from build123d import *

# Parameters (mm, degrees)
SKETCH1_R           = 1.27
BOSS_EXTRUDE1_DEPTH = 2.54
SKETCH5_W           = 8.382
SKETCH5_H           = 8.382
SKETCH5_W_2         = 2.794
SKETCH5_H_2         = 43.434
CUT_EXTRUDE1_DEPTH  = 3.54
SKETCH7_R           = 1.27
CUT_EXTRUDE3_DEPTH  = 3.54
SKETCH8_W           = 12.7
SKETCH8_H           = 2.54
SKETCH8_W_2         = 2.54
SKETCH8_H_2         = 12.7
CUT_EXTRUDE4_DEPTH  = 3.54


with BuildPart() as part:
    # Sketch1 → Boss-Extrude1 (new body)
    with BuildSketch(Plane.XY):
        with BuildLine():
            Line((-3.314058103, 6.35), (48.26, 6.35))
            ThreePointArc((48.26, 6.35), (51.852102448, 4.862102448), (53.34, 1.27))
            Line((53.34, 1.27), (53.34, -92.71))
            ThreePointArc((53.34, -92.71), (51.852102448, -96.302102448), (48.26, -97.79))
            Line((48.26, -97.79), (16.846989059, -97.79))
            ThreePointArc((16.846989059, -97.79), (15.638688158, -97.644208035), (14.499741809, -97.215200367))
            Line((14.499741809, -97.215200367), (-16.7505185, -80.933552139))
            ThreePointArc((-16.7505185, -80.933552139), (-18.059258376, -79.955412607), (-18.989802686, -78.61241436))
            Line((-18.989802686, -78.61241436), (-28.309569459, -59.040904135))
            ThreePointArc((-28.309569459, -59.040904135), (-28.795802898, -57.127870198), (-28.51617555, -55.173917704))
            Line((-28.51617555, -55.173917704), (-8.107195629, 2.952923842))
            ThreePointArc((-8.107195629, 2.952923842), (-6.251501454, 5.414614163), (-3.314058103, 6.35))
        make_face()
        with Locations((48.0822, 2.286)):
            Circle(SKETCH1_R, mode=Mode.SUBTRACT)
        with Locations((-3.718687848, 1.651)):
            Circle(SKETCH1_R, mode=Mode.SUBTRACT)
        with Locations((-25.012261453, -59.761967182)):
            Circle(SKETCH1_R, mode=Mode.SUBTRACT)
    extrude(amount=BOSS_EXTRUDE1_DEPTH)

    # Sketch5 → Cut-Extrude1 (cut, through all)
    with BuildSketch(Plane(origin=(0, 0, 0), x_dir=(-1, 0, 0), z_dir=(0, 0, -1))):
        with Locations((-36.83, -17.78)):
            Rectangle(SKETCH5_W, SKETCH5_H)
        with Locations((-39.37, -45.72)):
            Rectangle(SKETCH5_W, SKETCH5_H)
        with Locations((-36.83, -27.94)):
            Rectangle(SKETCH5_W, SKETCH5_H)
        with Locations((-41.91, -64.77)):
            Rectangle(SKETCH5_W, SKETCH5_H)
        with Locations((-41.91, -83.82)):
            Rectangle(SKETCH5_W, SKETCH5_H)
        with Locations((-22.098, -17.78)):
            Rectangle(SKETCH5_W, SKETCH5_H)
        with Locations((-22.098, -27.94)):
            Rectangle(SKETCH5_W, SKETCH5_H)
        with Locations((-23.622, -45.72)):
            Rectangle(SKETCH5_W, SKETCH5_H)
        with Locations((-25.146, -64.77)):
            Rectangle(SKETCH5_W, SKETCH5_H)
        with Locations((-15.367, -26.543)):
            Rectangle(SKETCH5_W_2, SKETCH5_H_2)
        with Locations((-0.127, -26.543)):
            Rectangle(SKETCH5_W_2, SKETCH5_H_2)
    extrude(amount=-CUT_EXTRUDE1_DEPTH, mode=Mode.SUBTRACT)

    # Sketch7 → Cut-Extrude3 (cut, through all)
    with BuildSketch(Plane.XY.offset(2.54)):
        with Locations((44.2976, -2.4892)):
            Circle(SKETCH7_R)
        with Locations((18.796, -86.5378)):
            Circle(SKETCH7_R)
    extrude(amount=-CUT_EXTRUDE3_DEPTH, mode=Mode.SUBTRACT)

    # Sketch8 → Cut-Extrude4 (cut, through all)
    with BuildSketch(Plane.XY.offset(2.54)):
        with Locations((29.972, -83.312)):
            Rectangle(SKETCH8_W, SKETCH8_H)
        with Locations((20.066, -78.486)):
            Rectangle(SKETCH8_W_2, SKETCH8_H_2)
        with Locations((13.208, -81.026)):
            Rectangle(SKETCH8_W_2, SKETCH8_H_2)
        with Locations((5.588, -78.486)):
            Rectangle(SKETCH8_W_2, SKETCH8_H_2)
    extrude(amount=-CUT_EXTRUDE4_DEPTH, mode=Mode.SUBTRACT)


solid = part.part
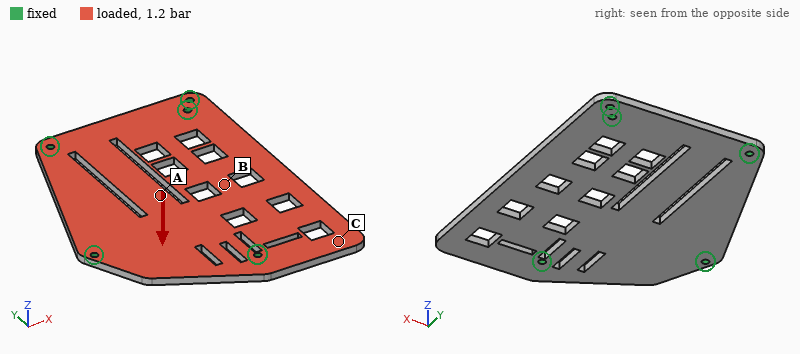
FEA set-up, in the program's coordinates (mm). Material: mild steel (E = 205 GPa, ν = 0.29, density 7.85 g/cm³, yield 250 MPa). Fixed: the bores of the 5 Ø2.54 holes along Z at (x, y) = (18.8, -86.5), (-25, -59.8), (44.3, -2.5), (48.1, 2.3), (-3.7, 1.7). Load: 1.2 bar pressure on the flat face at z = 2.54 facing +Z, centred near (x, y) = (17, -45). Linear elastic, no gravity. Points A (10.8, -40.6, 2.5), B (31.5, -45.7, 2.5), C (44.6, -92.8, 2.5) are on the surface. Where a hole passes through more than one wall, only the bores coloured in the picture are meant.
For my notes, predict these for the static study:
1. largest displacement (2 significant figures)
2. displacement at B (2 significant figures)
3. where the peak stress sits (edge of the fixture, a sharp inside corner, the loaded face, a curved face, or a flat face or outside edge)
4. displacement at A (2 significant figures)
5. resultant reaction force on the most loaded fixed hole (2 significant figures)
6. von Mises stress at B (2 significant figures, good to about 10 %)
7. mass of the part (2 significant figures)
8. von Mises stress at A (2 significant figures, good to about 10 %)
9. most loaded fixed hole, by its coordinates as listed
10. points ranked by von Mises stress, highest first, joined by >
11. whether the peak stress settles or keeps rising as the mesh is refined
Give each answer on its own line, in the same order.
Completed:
0.17 mm
0.11 mm
edge of the fixture
0.080 mm
340 N
58 MPa
120 g
33 MPa
(44.3, -2.5)
B > A > C
keeps rising
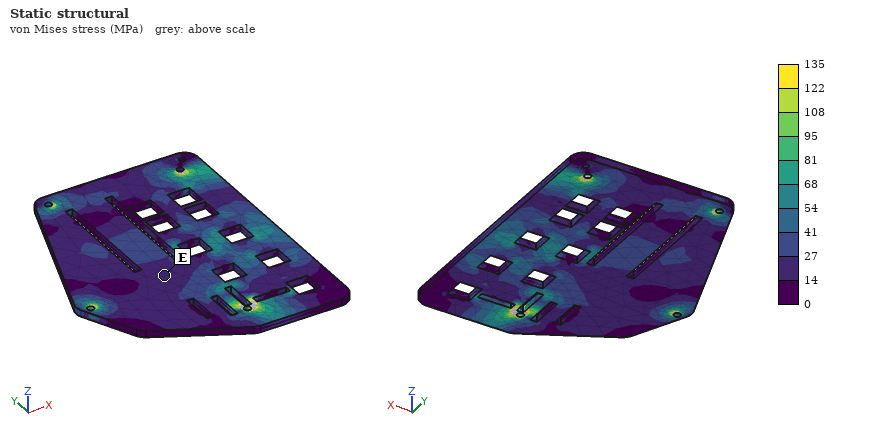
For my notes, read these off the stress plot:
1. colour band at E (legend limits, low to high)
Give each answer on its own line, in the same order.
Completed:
14 to 27 MPa
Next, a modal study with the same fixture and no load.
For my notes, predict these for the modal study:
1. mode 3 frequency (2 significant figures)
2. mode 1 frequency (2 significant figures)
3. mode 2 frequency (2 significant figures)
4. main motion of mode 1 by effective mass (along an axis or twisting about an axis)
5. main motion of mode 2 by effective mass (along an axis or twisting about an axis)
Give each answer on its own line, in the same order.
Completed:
2700 Hz
1200 Hz
1900 Hz
along Z
along Z
